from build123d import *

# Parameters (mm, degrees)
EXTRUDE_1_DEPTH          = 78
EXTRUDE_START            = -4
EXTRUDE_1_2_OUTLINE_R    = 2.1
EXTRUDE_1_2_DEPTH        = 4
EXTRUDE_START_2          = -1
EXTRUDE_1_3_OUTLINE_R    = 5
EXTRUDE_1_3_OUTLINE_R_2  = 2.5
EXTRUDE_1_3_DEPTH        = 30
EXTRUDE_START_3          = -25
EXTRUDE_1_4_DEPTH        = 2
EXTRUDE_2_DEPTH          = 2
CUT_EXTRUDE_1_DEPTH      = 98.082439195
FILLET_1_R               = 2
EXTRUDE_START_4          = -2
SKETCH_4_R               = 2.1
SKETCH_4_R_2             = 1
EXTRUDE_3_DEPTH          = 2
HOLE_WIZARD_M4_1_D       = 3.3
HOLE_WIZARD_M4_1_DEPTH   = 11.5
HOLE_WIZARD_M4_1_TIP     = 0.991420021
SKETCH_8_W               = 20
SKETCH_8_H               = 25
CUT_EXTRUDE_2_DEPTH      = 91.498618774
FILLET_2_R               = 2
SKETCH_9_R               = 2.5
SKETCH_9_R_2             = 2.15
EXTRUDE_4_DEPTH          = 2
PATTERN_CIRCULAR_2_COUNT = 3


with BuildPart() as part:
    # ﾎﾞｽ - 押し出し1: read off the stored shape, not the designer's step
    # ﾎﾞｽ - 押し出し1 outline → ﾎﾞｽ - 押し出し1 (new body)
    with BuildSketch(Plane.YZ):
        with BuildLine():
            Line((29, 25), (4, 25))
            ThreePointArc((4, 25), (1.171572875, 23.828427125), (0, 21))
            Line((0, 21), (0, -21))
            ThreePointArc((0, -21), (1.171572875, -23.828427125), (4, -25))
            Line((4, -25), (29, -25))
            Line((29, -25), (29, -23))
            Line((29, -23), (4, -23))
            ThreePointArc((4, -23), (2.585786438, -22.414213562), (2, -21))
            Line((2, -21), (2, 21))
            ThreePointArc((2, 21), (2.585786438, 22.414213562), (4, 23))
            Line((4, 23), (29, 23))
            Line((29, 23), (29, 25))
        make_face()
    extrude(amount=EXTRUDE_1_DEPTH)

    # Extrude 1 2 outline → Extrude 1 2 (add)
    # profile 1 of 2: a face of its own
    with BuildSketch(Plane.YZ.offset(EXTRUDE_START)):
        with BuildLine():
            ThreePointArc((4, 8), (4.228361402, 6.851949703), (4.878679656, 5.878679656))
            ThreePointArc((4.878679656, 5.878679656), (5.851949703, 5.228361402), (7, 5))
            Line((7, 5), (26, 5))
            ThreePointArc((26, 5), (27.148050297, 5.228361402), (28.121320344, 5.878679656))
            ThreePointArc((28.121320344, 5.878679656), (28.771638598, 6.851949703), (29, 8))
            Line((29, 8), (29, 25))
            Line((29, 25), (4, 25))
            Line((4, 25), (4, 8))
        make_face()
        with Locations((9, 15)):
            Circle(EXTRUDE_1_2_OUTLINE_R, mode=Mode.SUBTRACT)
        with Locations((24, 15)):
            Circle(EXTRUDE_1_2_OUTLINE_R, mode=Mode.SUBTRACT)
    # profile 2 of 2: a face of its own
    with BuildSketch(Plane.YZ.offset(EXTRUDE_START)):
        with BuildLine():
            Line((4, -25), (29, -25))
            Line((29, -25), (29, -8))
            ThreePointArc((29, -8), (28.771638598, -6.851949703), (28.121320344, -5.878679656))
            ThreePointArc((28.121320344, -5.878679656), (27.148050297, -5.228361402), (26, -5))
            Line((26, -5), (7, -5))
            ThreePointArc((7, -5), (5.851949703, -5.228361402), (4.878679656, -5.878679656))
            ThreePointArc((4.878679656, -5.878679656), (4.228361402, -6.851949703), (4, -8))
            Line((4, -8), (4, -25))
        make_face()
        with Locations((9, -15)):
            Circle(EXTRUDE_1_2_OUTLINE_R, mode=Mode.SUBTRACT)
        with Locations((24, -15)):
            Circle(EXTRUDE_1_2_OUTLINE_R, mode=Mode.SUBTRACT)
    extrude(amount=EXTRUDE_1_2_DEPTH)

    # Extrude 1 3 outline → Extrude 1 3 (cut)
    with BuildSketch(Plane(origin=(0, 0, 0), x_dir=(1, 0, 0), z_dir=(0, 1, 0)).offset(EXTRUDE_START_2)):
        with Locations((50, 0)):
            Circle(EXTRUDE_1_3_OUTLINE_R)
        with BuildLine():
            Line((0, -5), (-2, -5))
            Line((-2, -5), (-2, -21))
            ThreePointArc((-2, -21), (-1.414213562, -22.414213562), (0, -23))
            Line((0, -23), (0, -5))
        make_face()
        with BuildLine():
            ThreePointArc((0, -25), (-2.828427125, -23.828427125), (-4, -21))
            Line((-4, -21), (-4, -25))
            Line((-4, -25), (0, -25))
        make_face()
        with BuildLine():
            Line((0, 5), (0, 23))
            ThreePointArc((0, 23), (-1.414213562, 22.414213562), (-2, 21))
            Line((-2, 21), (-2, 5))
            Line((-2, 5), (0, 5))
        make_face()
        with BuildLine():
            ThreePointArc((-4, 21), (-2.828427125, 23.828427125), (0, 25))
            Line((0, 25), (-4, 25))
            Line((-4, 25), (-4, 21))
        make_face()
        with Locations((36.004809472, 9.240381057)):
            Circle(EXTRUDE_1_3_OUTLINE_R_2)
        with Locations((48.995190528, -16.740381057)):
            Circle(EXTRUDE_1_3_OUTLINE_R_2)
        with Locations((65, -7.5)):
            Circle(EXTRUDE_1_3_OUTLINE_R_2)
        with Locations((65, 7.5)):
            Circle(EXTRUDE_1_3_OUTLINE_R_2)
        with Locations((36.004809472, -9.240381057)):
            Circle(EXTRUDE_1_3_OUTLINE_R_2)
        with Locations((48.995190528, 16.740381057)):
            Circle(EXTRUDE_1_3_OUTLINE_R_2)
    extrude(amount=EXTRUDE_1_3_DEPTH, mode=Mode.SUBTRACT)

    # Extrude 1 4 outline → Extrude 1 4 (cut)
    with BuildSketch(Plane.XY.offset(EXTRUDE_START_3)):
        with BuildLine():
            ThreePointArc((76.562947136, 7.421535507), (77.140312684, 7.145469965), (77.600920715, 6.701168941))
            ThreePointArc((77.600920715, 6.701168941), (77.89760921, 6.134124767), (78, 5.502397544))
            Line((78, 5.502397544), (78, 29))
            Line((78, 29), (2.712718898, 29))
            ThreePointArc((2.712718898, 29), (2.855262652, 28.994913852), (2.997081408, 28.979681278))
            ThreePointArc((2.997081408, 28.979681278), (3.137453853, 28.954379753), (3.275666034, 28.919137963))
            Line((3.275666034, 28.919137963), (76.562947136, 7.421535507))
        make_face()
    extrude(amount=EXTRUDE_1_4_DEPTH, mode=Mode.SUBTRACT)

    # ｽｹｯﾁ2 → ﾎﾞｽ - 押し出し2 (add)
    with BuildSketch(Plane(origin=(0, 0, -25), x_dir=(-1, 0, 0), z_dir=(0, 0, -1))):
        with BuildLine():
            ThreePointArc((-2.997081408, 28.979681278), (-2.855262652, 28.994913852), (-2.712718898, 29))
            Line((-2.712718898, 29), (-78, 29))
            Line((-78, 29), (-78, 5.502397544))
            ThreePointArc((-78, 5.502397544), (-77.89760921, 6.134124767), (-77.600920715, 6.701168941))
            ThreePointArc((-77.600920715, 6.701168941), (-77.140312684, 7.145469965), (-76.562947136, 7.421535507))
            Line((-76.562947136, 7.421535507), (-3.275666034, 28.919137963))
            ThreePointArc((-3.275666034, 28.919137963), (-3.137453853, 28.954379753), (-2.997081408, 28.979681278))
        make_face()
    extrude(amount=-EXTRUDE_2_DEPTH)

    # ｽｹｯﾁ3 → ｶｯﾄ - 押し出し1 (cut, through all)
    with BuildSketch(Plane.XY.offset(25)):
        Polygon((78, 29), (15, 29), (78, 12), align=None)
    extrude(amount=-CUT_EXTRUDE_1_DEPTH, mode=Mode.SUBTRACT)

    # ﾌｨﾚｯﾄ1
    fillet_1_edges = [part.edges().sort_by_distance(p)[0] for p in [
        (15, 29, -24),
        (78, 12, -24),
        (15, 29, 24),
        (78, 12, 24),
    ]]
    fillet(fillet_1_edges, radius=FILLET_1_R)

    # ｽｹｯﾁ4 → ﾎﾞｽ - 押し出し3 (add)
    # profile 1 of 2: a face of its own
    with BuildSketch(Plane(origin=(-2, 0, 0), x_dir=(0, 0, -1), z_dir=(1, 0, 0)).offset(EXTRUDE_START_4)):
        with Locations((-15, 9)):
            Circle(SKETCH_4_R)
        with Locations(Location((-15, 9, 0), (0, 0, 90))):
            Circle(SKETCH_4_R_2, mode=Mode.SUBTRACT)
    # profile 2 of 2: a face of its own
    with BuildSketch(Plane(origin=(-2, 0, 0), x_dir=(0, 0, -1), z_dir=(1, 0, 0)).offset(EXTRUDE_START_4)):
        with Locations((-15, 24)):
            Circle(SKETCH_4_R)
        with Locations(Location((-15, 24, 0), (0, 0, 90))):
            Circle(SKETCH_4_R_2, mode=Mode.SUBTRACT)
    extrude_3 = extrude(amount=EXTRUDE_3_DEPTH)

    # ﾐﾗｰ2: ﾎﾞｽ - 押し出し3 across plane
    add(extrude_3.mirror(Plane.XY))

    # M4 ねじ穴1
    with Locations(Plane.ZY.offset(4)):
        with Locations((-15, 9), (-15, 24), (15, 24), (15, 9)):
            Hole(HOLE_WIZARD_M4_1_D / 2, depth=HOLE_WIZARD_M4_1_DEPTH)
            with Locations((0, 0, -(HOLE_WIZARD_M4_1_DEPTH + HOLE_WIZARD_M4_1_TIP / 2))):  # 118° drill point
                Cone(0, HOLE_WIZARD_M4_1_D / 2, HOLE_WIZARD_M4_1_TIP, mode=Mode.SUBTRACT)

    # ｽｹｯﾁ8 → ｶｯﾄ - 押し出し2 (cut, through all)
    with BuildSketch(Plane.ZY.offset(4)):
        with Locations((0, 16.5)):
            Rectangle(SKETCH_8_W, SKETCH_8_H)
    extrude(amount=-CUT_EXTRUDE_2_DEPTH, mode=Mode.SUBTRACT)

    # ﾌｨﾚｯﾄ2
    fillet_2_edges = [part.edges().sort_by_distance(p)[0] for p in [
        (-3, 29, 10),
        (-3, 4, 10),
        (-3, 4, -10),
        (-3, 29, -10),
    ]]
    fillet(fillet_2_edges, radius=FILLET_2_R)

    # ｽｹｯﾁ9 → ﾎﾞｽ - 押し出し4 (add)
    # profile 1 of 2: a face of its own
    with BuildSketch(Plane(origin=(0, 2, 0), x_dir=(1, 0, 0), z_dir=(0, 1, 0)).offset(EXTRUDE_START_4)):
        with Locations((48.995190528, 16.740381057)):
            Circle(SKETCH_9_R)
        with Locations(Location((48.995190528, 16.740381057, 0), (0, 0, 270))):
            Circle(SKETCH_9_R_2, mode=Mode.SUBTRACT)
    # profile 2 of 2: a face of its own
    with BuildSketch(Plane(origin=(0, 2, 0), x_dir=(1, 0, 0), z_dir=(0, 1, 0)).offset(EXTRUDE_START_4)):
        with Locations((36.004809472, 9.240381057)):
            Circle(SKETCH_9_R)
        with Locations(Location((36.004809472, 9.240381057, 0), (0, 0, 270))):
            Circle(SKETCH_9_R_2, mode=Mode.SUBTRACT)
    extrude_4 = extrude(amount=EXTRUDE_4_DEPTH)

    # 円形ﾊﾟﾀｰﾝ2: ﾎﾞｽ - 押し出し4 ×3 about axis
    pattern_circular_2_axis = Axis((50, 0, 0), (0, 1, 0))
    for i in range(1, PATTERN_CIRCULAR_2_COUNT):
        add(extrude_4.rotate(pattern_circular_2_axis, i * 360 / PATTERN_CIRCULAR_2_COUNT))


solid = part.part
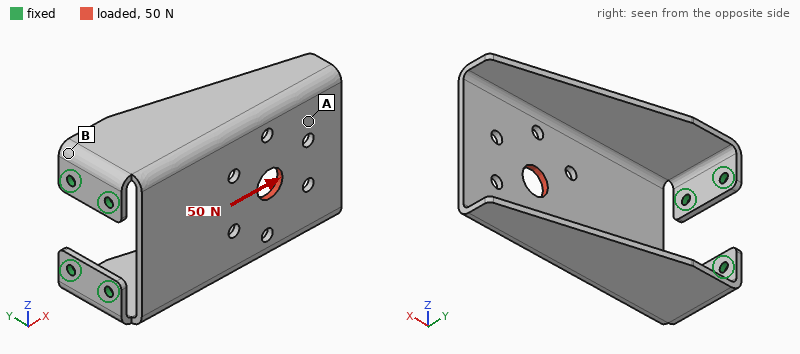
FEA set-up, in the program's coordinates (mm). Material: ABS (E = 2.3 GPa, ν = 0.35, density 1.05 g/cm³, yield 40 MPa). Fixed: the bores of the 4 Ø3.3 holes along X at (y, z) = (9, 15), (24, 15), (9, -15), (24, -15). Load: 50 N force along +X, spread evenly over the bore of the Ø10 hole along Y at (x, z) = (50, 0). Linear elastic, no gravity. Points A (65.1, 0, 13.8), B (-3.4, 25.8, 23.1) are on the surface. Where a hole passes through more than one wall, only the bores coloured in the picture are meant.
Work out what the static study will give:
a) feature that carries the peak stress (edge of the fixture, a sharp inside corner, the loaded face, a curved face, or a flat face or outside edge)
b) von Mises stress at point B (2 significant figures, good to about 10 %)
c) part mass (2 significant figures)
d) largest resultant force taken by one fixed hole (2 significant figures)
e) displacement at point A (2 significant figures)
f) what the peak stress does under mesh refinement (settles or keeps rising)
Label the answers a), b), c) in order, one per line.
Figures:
a) edge of the fixture
b) 3.6 MPa
c) 16 g
d) 38 N
e) 0.87 mm
f) keeps rising
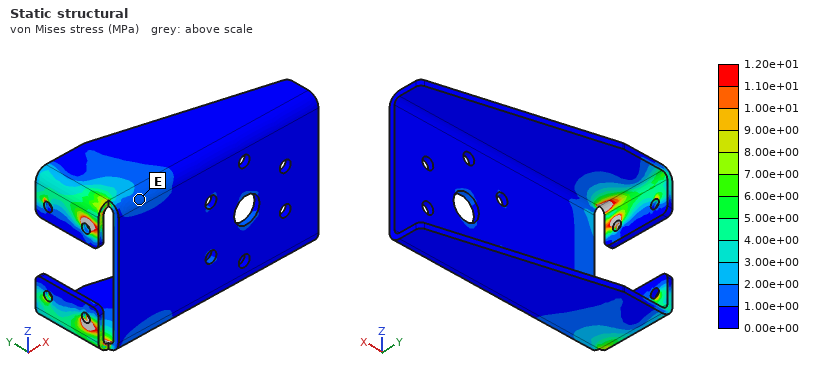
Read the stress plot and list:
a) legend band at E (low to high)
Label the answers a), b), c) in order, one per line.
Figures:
a) 1.00e+00 to 2.00e+00 MPa
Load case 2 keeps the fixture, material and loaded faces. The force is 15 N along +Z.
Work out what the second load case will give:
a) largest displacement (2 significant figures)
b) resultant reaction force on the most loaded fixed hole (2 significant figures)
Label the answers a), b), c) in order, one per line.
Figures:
a) 1.1 mm
b) 19 N
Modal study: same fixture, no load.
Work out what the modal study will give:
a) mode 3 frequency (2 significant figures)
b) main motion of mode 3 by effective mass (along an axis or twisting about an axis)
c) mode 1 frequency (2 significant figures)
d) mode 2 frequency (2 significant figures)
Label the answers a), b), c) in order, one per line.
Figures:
a) 530 Hz
b) along Z
c) 210 Hz
d) 210 Hz
